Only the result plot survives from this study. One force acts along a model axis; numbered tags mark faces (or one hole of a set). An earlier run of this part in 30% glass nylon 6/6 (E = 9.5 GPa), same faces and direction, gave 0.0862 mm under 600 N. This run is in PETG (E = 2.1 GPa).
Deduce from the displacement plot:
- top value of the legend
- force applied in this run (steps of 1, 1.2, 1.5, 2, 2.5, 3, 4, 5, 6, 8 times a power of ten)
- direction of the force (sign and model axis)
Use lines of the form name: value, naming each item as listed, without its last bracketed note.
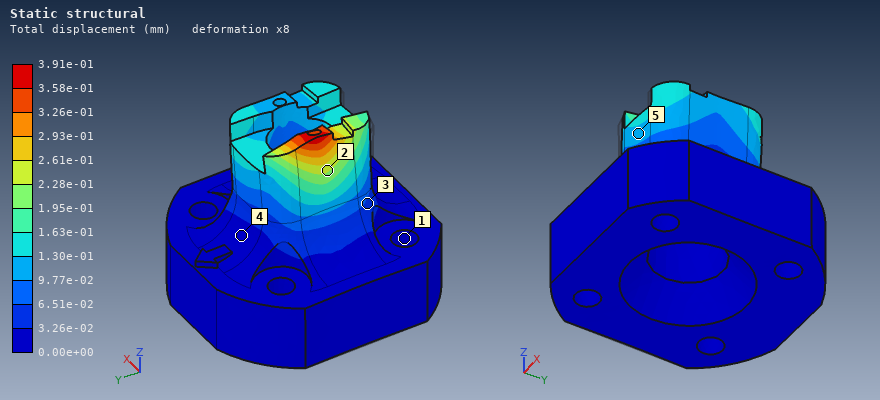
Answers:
top value of the legend: 3.91e-01 mm
force applied in this run: 600 N
direction of the force: +X
